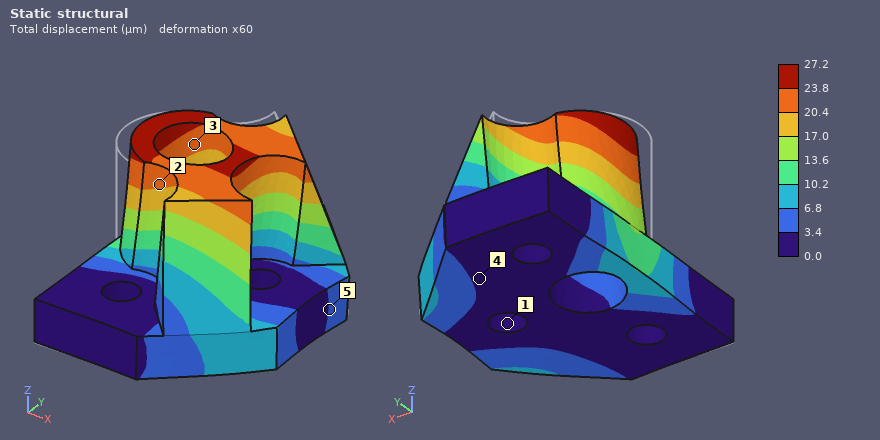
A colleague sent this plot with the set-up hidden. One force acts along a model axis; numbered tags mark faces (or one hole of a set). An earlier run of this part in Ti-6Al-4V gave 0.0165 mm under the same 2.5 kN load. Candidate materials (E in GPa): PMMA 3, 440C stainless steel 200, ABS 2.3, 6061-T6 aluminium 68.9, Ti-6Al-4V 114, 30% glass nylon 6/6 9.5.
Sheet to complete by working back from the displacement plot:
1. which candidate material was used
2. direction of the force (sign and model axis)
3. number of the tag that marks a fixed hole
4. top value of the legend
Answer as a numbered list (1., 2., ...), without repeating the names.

1. 6061-T6 aluminium
2. +X
3. 1
4. 27.2 µm
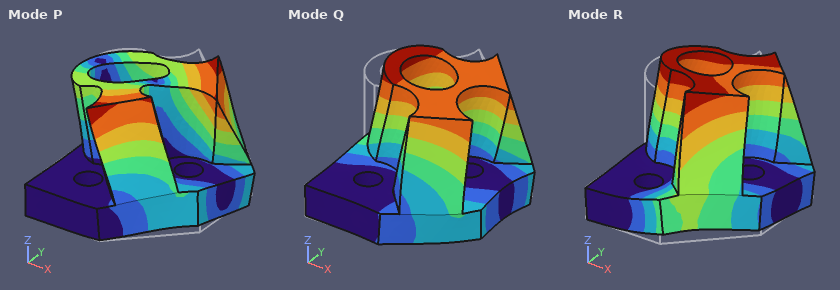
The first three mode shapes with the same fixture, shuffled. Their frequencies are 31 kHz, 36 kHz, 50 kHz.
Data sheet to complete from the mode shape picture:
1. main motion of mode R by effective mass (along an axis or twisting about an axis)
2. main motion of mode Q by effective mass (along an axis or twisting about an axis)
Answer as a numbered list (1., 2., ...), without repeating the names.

1. along Y
2. along X
